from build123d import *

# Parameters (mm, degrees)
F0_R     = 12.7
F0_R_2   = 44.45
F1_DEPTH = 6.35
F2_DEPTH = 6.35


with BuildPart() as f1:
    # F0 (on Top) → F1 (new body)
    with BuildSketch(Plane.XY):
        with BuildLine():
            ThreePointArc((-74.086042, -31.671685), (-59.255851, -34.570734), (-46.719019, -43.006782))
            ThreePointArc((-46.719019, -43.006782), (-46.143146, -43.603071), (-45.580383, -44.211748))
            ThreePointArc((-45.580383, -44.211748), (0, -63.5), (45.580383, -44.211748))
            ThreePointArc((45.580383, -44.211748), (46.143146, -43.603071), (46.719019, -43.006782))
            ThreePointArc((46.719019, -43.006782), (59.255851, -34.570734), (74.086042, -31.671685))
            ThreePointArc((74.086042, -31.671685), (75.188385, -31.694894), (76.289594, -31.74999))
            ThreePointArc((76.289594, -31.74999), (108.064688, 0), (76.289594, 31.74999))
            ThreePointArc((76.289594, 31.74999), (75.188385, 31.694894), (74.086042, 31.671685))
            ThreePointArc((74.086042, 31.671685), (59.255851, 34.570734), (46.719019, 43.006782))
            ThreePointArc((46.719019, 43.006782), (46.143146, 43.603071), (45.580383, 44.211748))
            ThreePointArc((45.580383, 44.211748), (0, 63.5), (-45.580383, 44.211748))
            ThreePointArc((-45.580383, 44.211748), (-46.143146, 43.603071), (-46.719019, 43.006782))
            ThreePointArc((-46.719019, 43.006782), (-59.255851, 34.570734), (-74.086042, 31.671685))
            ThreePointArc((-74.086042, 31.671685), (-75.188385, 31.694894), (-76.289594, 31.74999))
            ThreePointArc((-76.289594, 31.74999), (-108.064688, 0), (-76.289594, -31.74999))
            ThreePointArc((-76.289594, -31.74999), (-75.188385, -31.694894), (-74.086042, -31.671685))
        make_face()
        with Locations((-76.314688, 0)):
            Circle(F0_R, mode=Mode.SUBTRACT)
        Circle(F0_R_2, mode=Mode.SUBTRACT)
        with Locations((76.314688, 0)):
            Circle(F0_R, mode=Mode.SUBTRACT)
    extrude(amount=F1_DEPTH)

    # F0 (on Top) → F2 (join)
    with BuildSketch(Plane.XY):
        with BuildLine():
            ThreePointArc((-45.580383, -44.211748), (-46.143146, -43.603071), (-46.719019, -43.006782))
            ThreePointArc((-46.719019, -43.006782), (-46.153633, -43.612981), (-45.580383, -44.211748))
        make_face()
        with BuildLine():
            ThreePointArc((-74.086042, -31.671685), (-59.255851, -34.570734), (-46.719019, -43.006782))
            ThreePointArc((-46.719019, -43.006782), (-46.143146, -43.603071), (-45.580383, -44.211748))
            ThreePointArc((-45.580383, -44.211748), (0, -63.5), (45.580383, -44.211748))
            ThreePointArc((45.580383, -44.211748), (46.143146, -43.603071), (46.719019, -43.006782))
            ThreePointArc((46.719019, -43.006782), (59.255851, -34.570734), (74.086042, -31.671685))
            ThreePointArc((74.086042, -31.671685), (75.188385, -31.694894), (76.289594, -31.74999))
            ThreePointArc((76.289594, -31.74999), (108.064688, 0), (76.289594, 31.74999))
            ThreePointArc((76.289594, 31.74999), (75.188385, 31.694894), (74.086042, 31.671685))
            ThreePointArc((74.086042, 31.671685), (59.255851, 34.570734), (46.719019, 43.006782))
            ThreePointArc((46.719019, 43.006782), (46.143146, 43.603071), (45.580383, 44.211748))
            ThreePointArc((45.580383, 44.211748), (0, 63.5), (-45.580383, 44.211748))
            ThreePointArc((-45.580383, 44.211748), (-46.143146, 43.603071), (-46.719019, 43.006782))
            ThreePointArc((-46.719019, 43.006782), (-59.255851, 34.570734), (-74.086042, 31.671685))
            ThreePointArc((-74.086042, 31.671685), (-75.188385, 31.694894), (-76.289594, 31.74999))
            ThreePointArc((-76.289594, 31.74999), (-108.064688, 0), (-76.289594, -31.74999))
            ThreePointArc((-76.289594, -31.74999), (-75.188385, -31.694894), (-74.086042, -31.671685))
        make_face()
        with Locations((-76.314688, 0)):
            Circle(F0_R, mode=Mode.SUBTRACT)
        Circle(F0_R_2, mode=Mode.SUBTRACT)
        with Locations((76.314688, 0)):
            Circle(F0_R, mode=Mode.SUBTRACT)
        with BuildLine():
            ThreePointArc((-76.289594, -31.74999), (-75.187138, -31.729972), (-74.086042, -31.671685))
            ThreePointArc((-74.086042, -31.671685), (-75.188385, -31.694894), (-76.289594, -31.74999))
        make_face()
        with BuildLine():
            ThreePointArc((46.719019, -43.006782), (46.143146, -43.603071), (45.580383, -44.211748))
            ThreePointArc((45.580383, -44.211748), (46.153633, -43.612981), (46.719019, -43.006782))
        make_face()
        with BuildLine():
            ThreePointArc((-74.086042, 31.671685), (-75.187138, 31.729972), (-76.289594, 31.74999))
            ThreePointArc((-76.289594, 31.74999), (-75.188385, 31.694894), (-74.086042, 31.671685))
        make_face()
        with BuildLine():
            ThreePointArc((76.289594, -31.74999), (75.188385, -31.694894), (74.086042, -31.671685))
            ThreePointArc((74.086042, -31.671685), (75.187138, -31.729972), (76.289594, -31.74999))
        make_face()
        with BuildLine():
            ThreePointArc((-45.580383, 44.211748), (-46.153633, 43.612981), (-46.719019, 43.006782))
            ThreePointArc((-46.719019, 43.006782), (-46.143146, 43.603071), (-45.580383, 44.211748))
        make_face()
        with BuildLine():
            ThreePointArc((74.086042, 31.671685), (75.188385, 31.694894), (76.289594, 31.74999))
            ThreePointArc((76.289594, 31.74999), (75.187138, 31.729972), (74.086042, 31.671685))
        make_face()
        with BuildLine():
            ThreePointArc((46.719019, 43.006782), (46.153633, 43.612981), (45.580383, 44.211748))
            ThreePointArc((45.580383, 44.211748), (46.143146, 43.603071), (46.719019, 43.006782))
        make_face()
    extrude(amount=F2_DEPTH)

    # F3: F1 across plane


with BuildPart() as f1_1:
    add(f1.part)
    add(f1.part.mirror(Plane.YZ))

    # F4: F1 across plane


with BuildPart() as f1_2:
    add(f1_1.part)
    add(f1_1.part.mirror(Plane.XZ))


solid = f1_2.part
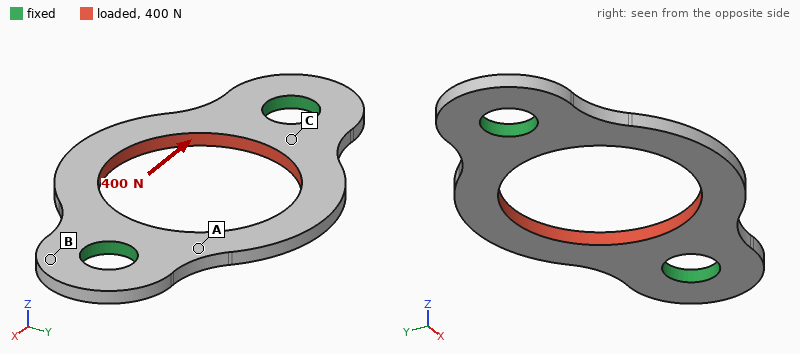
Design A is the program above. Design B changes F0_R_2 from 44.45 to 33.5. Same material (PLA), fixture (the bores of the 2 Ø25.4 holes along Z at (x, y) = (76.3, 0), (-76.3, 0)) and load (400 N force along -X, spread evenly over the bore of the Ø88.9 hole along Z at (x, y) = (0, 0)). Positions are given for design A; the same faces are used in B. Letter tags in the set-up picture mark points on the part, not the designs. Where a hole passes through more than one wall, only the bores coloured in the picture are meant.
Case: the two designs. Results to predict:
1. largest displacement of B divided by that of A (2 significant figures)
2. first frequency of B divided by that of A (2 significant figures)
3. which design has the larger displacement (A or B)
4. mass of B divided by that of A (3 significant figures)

0.56
0.99
A
1.25
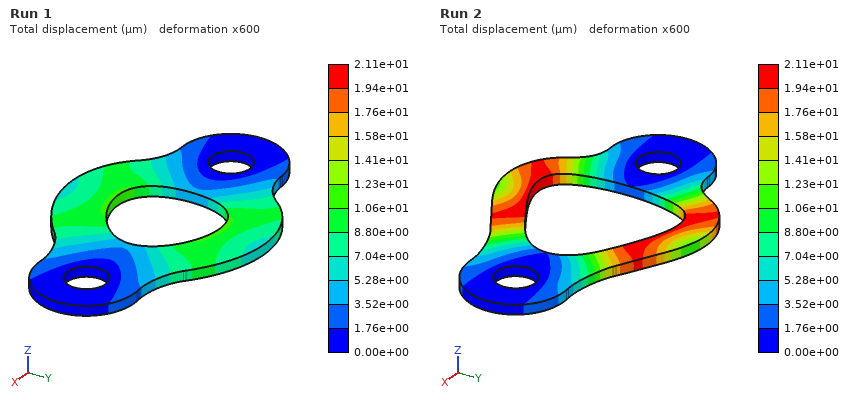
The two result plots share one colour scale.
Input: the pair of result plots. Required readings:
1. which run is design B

Run 1
